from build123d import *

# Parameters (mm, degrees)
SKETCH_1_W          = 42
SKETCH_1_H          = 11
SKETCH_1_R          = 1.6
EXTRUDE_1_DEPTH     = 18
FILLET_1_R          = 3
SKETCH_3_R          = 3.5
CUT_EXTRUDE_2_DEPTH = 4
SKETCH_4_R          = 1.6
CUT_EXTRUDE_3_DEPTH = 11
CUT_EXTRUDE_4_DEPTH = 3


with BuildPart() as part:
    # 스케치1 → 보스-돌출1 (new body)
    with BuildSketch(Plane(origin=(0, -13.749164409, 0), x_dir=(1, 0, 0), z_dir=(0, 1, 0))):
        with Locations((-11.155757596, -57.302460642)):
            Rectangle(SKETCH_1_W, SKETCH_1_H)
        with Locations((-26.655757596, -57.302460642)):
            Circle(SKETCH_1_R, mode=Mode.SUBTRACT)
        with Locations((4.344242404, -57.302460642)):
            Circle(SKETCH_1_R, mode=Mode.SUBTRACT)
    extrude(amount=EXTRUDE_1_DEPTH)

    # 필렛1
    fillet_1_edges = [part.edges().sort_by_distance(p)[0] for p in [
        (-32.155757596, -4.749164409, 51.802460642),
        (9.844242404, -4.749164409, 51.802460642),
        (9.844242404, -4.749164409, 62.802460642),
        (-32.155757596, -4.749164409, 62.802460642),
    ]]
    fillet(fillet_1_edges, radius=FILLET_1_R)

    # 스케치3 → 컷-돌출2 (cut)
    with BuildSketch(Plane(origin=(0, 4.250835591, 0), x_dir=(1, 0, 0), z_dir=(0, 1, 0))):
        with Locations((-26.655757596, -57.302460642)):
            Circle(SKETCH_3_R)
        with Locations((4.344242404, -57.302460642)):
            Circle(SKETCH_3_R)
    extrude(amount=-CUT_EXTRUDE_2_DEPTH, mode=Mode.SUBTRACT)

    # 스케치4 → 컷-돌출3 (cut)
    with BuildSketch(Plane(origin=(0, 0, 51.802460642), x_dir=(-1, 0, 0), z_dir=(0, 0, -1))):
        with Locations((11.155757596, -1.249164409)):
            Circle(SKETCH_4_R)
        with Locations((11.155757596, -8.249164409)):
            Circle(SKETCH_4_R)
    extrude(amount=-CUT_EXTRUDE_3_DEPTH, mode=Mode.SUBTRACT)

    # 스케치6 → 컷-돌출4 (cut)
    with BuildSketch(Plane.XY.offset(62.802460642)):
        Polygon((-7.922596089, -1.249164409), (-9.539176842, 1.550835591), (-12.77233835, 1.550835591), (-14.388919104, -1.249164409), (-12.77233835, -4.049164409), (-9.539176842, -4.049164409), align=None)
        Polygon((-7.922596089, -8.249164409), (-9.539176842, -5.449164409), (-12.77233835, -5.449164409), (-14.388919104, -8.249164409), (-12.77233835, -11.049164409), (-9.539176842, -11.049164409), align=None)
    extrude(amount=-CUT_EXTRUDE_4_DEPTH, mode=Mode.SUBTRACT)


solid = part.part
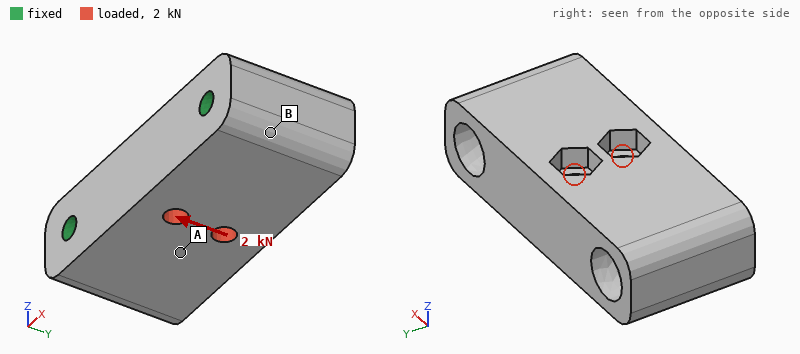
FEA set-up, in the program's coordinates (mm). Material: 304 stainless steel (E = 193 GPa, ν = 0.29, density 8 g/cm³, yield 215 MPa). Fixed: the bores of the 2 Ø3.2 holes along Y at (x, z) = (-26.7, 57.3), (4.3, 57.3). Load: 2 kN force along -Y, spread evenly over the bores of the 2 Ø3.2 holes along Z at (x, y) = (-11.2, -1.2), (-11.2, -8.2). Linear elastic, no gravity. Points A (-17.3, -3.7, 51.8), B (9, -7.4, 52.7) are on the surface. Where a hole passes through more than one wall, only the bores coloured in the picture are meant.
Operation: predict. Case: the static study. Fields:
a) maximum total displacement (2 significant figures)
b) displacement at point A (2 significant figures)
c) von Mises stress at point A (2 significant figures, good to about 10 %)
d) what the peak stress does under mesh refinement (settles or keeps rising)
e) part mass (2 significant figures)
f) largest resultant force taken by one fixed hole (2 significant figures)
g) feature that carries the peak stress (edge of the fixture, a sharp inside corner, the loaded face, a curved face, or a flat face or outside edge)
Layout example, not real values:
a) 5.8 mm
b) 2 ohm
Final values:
a) 2.2 µm
b) 1.4 µm
c) 15 MPa
d) keeps rising
e) 59 g
f) 1.0 kN
g) edge of the fixture
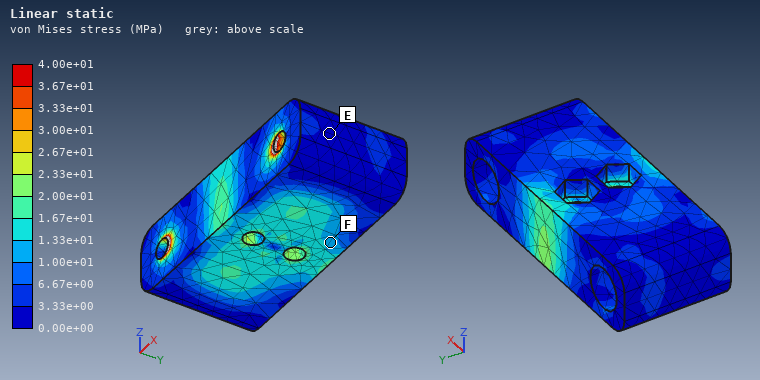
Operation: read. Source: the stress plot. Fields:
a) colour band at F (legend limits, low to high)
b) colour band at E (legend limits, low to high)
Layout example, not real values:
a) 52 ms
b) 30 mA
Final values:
a) 1.00e+01 to 1.33e+01 MPa
b) 0.00e+00 to 3.33e+00 MPa
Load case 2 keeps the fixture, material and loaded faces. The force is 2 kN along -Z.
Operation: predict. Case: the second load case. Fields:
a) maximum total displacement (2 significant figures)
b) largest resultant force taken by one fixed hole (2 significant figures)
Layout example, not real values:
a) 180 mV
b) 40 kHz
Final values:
a) 3.8 µm
b) 1.0 kN
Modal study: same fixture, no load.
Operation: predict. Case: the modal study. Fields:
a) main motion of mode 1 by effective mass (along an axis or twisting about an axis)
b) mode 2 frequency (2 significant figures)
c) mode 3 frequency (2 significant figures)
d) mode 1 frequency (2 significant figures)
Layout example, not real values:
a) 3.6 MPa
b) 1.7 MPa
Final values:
a) along Z
b) 38 kHz
c) 39 kHz
d) 27 kHz
